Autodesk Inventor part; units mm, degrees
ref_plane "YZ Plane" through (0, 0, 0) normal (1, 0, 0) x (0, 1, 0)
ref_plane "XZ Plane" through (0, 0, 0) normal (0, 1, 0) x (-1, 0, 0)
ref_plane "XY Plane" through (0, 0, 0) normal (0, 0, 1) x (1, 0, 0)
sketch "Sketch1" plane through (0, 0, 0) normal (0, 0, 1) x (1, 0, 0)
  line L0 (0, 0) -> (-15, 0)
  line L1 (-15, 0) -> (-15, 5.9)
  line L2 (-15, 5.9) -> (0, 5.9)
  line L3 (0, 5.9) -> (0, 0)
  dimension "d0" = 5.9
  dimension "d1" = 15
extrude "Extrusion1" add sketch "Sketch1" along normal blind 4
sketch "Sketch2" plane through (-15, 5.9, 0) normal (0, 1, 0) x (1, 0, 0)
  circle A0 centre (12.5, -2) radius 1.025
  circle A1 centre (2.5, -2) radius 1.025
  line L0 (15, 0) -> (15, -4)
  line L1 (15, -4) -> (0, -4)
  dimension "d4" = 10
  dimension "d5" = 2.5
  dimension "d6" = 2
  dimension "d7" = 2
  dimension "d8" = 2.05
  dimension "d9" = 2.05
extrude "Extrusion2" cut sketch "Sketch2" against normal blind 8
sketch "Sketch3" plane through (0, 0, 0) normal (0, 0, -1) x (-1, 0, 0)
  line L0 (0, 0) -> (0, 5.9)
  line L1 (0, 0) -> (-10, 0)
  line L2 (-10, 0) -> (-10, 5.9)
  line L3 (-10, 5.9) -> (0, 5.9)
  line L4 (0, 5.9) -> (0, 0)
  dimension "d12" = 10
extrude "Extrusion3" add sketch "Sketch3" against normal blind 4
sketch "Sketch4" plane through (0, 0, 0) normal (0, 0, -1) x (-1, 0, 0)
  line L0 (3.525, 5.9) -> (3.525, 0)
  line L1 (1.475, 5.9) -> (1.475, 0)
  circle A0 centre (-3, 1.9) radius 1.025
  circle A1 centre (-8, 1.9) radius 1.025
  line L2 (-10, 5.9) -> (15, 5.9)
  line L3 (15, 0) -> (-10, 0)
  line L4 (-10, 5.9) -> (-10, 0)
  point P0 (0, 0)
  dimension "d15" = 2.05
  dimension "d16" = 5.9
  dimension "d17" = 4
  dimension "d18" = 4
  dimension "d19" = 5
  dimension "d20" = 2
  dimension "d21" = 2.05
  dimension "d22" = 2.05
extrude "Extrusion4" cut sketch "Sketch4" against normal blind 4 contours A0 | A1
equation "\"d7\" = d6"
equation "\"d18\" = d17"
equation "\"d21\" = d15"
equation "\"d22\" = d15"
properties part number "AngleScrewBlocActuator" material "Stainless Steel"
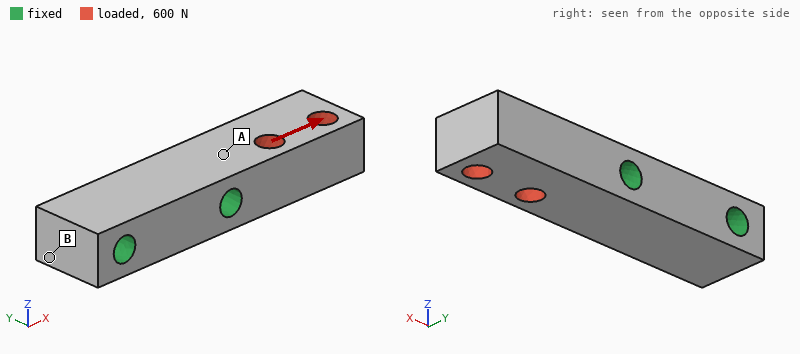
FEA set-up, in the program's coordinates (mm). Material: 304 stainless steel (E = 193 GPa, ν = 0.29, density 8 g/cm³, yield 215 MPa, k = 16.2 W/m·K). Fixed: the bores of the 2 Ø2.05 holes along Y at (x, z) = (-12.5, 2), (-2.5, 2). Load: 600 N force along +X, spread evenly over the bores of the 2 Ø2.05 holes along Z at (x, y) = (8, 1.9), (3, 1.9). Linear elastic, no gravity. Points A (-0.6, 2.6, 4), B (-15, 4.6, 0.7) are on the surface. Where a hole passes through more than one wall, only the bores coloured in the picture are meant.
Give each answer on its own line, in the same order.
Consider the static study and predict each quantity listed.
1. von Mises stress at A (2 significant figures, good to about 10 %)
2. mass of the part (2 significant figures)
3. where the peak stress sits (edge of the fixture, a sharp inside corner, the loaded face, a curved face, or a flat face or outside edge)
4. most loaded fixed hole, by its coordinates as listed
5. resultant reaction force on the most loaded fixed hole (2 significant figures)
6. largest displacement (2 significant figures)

17 MPa
4.2 g
the loaded face
(-2.5, 2)
590 N
4.4 µm
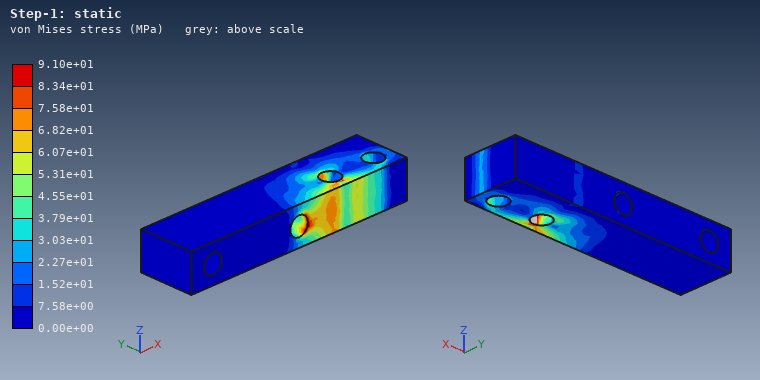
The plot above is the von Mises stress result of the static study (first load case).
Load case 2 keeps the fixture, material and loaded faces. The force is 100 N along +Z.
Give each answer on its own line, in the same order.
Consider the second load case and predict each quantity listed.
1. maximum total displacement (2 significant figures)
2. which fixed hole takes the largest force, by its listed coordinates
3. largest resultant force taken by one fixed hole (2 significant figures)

7.4 µm
(-2.5, 2)
110 N
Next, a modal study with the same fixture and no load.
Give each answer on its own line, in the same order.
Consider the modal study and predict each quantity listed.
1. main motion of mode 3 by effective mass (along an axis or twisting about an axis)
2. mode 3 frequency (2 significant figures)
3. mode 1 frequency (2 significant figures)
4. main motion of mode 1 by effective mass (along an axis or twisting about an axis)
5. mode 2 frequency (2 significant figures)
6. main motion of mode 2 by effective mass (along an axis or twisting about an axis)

twisting about X
53 kHz
19 kHz
along Z
28 kHz
along Y
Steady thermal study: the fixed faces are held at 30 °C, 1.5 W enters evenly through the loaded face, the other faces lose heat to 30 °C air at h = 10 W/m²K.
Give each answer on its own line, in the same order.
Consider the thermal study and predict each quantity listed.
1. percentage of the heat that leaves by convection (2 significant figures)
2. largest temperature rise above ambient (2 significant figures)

3.5 %
35 K
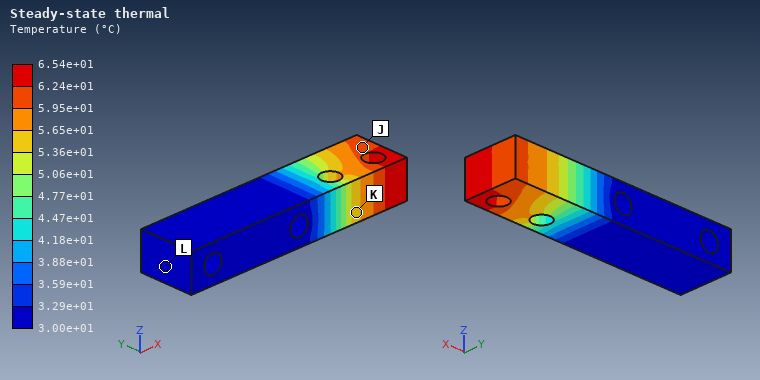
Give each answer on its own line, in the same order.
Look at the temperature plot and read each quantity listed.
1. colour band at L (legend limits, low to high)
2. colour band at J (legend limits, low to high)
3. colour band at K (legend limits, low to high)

3.00e+01 to 3.29e+01 °C
5.95e+01 to 6.24e+01 °C
5.36e+01 to 5.65e+01 °C
